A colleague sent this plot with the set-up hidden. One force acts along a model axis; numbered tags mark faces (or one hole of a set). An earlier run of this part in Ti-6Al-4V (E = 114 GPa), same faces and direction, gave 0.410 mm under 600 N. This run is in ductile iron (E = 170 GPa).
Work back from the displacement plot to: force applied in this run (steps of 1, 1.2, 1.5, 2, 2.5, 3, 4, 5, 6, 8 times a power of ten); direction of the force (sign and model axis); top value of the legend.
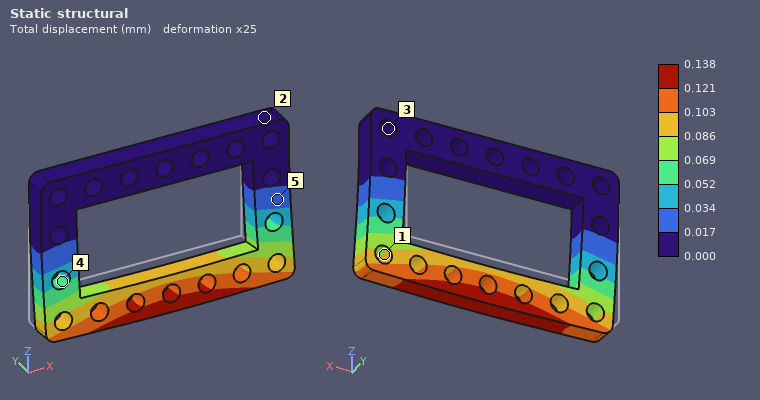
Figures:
300 N
-Y
0.138 mm
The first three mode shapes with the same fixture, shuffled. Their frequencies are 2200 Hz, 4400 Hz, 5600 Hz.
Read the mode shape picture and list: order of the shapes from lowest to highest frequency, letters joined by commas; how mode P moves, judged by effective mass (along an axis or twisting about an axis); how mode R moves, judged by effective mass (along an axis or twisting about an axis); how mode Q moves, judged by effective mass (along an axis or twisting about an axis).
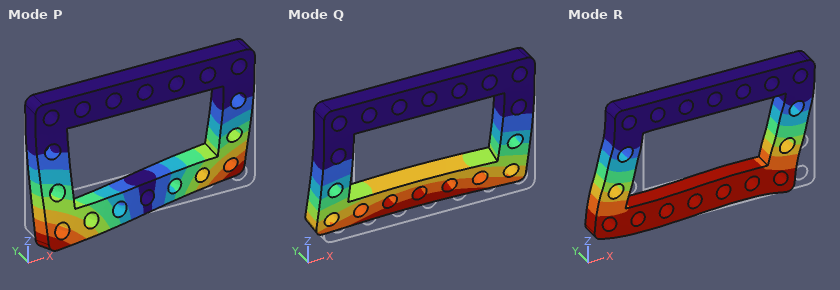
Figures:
Q, P, R
twisting about Z
along X
along Y
